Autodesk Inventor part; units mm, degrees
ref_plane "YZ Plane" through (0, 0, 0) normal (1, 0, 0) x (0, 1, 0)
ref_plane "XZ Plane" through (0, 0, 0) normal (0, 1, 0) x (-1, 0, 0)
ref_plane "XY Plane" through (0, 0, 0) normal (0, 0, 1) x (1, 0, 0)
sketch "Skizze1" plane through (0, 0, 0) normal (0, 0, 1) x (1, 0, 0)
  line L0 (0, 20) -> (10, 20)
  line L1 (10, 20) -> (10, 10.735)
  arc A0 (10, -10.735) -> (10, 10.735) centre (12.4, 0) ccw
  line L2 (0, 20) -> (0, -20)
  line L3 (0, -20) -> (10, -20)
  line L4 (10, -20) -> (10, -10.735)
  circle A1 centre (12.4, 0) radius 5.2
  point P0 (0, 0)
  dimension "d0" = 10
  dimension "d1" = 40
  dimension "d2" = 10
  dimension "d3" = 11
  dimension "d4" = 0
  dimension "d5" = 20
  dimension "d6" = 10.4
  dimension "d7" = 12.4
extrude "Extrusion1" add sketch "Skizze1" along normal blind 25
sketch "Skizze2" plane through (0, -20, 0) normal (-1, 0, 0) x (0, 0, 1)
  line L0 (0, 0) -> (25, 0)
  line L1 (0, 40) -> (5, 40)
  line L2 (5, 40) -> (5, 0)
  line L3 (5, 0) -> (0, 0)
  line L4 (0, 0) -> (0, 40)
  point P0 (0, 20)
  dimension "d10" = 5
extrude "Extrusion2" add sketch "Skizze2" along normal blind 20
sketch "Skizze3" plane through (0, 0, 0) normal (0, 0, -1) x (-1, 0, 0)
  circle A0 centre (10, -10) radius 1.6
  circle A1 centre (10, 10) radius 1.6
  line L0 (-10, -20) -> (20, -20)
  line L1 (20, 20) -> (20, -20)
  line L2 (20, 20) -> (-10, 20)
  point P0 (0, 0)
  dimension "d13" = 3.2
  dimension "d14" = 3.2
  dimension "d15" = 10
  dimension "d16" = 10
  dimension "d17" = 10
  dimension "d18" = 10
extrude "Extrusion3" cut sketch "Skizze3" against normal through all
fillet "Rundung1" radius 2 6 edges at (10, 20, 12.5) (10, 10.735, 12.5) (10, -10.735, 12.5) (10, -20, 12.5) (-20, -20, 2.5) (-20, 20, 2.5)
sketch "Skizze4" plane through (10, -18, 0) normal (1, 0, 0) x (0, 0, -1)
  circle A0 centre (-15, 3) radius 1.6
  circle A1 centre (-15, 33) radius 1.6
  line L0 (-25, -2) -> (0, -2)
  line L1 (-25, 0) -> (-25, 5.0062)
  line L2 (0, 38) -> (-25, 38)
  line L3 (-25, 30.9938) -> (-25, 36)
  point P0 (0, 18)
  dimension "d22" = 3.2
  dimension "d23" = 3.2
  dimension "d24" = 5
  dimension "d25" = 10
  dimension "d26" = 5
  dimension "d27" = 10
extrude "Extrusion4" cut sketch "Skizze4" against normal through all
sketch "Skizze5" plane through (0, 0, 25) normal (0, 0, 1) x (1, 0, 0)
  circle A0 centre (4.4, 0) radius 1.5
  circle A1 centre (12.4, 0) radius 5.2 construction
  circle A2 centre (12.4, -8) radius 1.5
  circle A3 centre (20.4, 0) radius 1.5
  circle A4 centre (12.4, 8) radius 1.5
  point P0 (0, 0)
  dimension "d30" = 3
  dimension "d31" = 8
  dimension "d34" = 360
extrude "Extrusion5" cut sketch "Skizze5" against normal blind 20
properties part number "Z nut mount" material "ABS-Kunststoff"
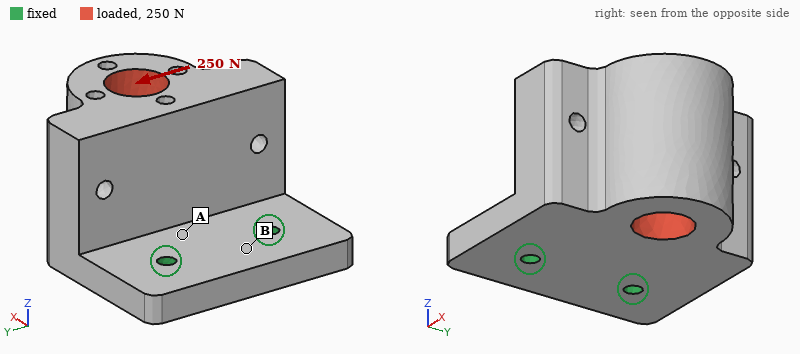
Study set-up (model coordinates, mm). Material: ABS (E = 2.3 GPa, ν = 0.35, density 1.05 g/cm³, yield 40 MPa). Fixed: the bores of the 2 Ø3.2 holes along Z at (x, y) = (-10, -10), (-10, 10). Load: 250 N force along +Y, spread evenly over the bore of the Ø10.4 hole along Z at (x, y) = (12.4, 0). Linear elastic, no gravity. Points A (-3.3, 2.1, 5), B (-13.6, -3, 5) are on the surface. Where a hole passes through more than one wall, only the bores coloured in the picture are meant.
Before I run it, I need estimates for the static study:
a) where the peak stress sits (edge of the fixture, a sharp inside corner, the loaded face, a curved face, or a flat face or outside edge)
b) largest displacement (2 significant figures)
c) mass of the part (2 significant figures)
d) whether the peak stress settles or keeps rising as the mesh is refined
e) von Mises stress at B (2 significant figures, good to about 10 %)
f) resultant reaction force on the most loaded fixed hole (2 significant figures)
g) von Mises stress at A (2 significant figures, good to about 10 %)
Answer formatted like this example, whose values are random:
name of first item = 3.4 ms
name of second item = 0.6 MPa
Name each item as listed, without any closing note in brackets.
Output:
where the peak stress sits = edge of the fixture
largest displacement = 0.21 mm
mass of the part = 18 g
whether the peak stress settles or keeps rising as the mesh is refined = keeps rising
von Mises stress at B = 2.2 MPa
resultant reaction force on the most loaded fixed hole = 300 N
von Mises stress at A = 7.0 MPa
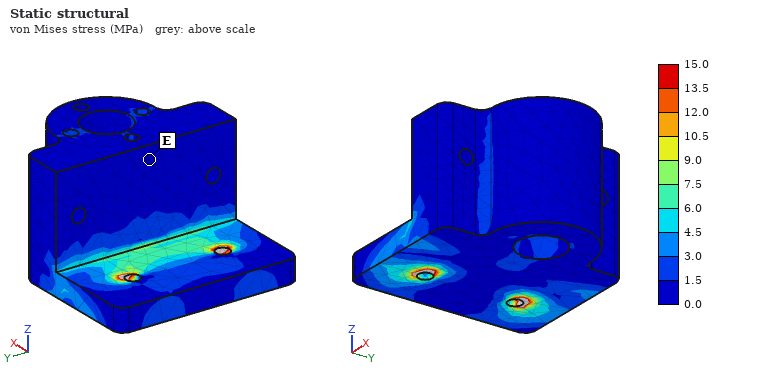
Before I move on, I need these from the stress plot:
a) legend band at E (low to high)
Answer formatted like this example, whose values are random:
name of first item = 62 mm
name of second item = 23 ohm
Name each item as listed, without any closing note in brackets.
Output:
legend band at E = 0.0 to 1.5 MPa
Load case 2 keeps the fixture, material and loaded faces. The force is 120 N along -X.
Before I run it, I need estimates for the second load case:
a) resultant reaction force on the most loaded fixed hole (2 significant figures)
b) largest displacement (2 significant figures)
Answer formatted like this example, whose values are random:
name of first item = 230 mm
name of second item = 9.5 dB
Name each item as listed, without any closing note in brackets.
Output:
resultant reaction force on the most loaded fixed hole = 61 N
largest displacement = 0.59 mm
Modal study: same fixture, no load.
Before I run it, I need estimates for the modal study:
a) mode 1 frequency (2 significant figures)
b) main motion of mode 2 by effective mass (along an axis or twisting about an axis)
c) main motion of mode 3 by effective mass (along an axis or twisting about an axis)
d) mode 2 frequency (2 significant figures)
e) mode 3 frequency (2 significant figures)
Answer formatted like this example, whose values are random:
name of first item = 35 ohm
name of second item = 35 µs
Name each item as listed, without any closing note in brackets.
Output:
mode 1 frequency = 600 Hz
main motion of mode 2 by effective mass = along Y
main motion of mode 3 by effective mass = along Y
mode 2 frequency = 1600 Hz
mode 3 frequency = 3000 Hz
